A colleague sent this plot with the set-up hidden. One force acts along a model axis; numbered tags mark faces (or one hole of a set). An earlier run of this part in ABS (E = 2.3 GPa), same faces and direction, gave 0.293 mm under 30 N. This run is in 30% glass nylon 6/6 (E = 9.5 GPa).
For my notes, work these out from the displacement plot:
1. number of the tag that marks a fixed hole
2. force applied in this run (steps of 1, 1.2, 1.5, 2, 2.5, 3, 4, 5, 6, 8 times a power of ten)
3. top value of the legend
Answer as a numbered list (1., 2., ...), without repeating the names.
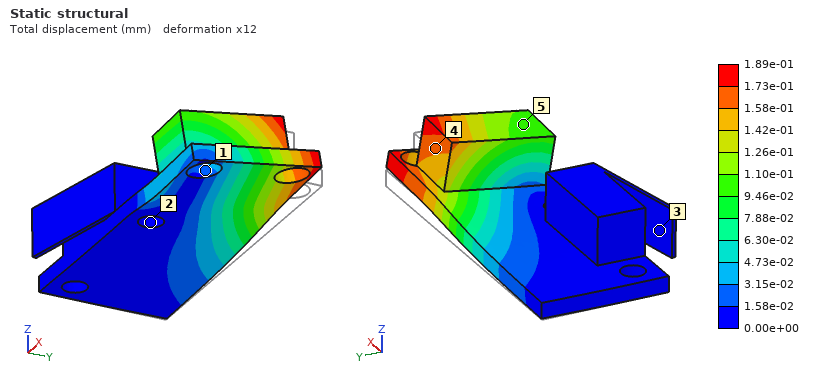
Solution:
1. 2
2. 80 N
3. 1.89e-01 mm
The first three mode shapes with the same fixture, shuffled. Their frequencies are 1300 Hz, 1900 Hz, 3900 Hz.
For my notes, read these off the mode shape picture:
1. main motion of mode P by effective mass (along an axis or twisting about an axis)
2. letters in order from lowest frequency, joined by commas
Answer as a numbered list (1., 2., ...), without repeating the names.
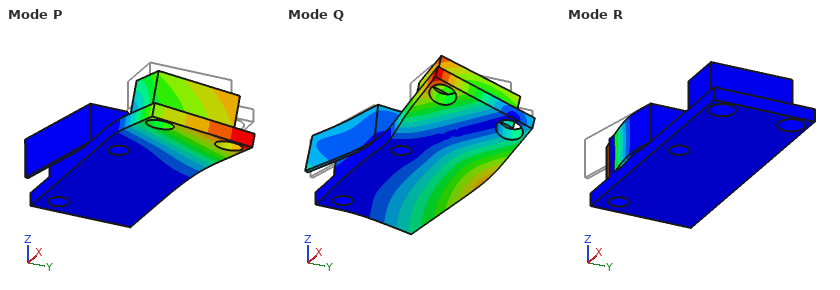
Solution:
1. along Z
2. R, P, Q
